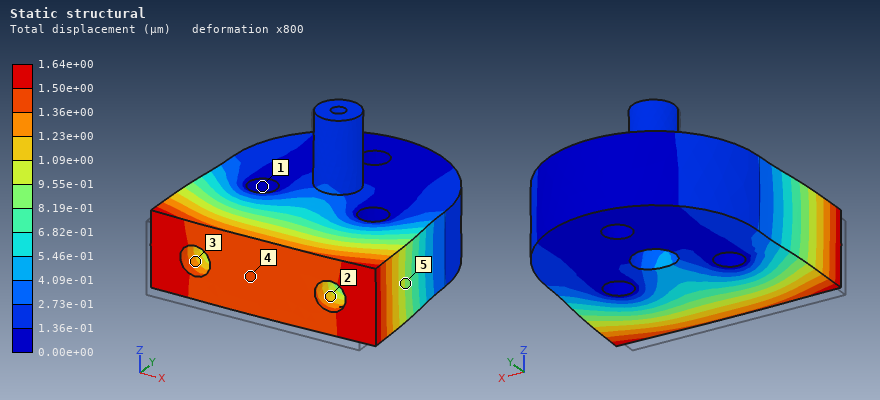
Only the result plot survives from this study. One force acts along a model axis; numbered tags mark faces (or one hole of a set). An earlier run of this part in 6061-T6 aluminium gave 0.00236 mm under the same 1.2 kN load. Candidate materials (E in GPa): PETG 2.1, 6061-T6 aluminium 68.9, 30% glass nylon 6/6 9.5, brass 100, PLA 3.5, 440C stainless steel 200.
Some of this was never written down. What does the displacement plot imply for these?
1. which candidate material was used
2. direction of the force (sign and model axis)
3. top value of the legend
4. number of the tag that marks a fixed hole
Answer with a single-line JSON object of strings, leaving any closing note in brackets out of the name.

{"which candidate material was used": "brass", "direction of the force": "+Y", "top value of the legend": "1.64e+00 µm", "number of the tag that marks a fixed hole": "1"}
